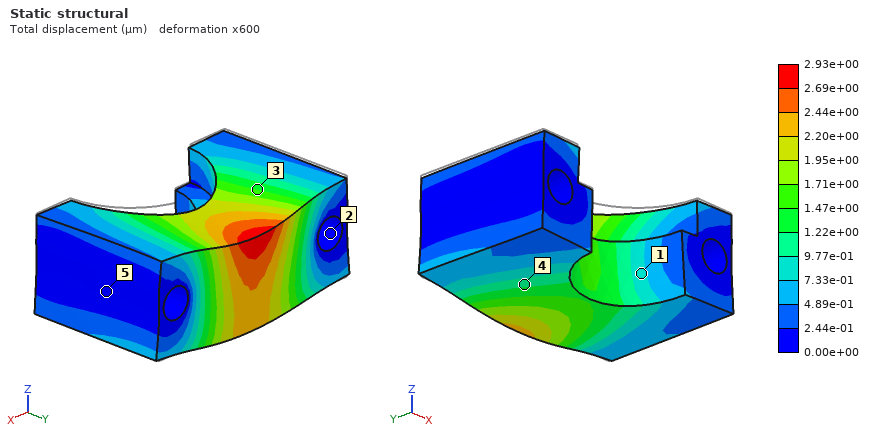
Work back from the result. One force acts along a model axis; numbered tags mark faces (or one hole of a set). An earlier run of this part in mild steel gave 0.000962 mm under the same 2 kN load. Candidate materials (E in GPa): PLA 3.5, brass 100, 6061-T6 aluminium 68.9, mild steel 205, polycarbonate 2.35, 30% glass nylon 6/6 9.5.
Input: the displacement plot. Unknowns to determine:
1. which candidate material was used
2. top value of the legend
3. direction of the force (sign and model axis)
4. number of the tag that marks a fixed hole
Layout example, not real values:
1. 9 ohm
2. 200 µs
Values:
1. 6061-T6 aluminium
2. 2.93e+00 µm
3. -Z
4. 2
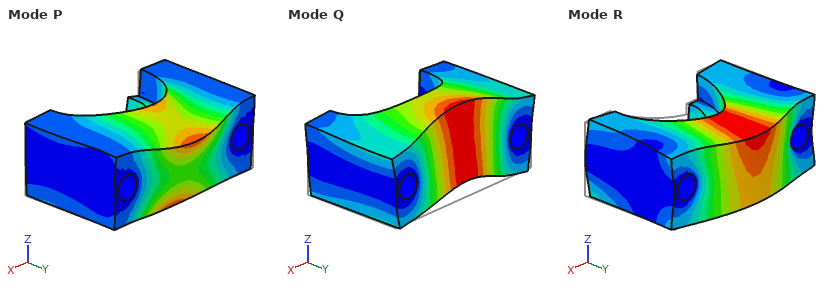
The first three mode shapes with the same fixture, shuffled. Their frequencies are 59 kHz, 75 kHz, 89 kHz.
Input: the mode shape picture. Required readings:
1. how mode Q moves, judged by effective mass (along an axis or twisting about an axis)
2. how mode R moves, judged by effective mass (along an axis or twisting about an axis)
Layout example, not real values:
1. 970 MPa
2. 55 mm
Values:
1. along Z
2. along Y
